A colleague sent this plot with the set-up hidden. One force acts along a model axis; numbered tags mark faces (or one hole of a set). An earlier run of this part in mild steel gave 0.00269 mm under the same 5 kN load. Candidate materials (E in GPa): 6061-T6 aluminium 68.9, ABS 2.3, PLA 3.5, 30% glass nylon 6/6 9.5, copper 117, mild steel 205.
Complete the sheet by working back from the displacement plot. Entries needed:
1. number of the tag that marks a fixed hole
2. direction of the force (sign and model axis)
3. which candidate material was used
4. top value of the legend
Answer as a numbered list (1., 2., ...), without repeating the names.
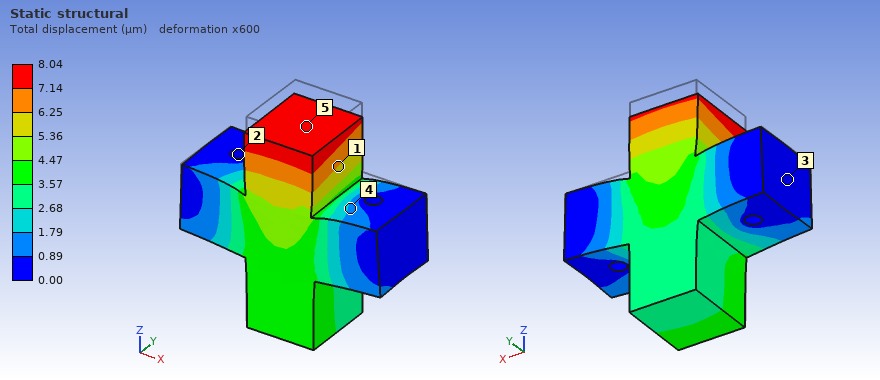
1. 2
2. -Z
3. 6061-T6 aluminium
4. 8.04 µm
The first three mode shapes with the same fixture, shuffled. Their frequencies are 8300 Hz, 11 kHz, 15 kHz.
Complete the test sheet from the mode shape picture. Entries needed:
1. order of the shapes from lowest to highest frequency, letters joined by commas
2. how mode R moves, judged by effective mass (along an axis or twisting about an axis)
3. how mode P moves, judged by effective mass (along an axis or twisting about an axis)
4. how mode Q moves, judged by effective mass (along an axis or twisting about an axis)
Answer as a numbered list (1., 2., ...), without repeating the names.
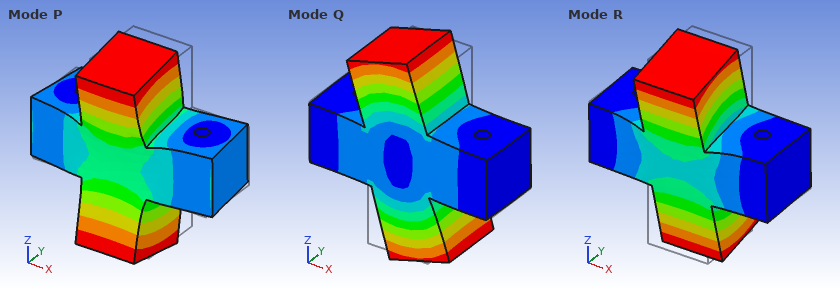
1. R, P, Q
2. twisting about X
3. along Y
4. twisting about Y
